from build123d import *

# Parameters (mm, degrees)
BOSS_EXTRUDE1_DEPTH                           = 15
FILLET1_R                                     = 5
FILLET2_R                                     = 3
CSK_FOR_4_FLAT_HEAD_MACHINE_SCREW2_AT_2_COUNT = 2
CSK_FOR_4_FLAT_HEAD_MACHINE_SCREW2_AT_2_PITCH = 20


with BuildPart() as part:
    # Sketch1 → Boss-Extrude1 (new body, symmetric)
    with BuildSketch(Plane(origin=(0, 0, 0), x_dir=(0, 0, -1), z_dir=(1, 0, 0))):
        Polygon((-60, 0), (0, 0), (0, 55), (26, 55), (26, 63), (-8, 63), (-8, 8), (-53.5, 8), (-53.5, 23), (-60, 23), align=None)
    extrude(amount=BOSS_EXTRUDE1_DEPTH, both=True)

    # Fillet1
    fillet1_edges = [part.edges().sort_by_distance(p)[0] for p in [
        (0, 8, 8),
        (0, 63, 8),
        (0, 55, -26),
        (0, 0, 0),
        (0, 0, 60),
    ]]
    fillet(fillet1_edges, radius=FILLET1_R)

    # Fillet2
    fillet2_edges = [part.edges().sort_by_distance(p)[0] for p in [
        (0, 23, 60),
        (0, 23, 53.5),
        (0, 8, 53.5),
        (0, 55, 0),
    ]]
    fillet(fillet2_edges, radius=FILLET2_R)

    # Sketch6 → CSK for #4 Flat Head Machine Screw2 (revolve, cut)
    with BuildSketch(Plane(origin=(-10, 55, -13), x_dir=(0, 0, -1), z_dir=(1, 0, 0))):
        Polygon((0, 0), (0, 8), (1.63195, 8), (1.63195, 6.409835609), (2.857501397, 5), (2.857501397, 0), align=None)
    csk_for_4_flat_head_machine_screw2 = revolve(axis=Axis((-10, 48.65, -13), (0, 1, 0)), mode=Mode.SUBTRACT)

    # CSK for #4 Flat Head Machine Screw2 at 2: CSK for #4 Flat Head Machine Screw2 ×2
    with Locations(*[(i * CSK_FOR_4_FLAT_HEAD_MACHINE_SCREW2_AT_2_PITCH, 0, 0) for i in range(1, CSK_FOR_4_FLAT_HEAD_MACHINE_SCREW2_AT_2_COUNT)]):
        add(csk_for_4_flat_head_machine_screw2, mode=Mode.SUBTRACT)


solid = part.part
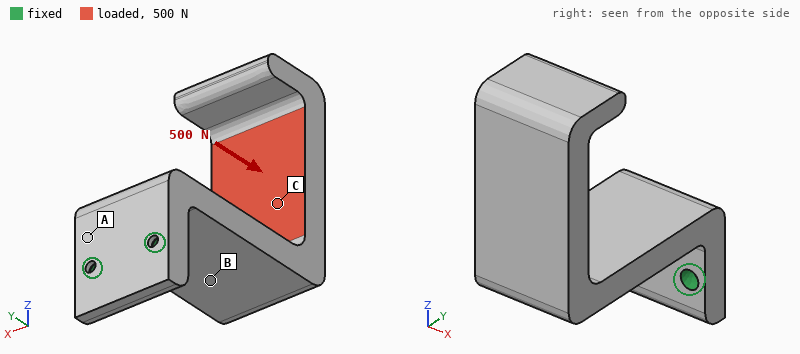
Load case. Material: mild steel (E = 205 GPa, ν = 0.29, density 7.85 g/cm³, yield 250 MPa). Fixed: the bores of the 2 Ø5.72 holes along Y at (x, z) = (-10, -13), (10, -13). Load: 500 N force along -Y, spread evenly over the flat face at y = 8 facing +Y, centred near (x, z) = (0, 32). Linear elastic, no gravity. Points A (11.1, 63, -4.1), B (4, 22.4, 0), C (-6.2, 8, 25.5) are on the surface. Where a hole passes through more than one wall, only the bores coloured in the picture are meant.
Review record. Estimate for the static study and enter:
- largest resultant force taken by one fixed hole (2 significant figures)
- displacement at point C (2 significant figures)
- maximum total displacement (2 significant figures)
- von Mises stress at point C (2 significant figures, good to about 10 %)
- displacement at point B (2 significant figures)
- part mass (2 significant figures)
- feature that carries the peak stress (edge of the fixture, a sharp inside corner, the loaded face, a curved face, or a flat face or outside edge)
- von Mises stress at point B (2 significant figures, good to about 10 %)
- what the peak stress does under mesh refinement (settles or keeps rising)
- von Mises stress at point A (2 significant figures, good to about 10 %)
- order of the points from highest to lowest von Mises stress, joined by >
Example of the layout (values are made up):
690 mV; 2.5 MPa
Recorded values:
290 N; 0.15 mm; 0.28 mm; 13 MPa; 0.072 mm; 280 g; edge of the fixture; 39 MPa; keeps rising; 55 MPa; A > B > C
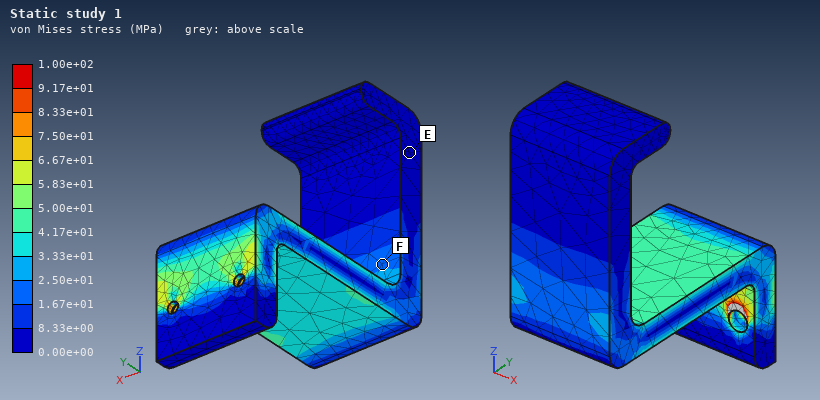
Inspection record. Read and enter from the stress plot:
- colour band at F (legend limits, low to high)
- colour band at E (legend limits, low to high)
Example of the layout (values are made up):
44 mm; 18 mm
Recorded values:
1.67e+01 to 2.50e+01 MPa; 0.00e+00 to 8.33e+00 MPa
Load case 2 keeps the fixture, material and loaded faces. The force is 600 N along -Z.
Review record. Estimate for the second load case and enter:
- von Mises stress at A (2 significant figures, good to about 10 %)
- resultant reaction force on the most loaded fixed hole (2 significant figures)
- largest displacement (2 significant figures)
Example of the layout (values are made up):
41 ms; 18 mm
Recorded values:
91 MPa; 390 N; 0.33 mm
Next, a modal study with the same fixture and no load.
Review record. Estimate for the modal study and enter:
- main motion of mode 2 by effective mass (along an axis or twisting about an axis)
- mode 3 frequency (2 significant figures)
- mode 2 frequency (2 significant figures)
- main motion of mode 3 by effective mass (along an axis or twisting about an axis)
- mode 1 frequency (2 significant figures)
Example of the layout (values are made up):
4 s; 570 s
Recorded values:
along X; 1600 Hz; 940 Hz; along Z; 510 Hz
